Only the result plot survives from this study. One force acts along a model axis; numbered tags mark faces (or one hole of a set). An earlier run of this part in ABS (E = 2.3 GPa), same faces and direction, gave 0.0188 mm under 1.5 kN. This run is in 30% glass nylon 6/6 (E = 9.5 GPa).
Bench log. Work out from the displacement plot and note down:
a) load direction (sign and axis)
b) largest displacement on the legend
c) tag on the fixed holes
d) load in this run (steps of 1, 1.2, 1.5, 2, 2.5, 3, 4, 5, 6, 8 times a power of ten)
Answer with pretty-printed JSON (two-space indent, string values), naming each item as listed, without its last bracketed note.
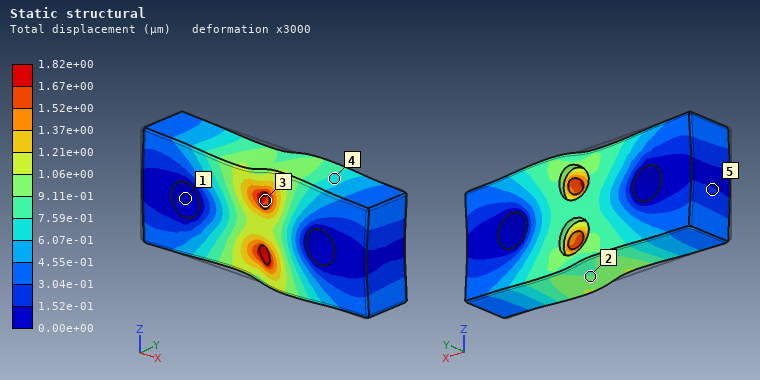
{
  "load direction": "+X",
  "largest displacement on the legend": "1.82e+00 µm",
  "tag on the fixed holes": "1",
  "load in this run": "600 N"
}
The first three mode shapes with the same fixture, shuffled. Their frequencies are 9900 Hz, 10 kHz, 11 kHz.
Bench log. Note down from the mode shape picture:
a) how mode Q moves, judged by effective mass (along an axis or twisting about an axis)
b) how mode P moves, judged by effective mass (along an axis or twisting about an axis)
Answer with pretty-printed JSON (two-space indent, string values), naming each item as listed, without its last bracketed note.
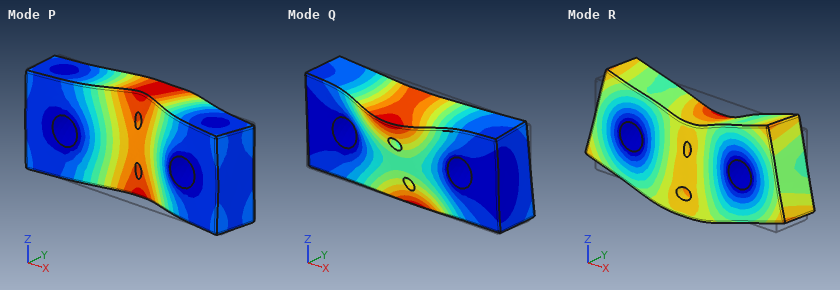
{
  "how mode Q moves, judged by effective mass": "twisting about X",
  "how mode P moves, judged by effective mass": "along Y"
}
